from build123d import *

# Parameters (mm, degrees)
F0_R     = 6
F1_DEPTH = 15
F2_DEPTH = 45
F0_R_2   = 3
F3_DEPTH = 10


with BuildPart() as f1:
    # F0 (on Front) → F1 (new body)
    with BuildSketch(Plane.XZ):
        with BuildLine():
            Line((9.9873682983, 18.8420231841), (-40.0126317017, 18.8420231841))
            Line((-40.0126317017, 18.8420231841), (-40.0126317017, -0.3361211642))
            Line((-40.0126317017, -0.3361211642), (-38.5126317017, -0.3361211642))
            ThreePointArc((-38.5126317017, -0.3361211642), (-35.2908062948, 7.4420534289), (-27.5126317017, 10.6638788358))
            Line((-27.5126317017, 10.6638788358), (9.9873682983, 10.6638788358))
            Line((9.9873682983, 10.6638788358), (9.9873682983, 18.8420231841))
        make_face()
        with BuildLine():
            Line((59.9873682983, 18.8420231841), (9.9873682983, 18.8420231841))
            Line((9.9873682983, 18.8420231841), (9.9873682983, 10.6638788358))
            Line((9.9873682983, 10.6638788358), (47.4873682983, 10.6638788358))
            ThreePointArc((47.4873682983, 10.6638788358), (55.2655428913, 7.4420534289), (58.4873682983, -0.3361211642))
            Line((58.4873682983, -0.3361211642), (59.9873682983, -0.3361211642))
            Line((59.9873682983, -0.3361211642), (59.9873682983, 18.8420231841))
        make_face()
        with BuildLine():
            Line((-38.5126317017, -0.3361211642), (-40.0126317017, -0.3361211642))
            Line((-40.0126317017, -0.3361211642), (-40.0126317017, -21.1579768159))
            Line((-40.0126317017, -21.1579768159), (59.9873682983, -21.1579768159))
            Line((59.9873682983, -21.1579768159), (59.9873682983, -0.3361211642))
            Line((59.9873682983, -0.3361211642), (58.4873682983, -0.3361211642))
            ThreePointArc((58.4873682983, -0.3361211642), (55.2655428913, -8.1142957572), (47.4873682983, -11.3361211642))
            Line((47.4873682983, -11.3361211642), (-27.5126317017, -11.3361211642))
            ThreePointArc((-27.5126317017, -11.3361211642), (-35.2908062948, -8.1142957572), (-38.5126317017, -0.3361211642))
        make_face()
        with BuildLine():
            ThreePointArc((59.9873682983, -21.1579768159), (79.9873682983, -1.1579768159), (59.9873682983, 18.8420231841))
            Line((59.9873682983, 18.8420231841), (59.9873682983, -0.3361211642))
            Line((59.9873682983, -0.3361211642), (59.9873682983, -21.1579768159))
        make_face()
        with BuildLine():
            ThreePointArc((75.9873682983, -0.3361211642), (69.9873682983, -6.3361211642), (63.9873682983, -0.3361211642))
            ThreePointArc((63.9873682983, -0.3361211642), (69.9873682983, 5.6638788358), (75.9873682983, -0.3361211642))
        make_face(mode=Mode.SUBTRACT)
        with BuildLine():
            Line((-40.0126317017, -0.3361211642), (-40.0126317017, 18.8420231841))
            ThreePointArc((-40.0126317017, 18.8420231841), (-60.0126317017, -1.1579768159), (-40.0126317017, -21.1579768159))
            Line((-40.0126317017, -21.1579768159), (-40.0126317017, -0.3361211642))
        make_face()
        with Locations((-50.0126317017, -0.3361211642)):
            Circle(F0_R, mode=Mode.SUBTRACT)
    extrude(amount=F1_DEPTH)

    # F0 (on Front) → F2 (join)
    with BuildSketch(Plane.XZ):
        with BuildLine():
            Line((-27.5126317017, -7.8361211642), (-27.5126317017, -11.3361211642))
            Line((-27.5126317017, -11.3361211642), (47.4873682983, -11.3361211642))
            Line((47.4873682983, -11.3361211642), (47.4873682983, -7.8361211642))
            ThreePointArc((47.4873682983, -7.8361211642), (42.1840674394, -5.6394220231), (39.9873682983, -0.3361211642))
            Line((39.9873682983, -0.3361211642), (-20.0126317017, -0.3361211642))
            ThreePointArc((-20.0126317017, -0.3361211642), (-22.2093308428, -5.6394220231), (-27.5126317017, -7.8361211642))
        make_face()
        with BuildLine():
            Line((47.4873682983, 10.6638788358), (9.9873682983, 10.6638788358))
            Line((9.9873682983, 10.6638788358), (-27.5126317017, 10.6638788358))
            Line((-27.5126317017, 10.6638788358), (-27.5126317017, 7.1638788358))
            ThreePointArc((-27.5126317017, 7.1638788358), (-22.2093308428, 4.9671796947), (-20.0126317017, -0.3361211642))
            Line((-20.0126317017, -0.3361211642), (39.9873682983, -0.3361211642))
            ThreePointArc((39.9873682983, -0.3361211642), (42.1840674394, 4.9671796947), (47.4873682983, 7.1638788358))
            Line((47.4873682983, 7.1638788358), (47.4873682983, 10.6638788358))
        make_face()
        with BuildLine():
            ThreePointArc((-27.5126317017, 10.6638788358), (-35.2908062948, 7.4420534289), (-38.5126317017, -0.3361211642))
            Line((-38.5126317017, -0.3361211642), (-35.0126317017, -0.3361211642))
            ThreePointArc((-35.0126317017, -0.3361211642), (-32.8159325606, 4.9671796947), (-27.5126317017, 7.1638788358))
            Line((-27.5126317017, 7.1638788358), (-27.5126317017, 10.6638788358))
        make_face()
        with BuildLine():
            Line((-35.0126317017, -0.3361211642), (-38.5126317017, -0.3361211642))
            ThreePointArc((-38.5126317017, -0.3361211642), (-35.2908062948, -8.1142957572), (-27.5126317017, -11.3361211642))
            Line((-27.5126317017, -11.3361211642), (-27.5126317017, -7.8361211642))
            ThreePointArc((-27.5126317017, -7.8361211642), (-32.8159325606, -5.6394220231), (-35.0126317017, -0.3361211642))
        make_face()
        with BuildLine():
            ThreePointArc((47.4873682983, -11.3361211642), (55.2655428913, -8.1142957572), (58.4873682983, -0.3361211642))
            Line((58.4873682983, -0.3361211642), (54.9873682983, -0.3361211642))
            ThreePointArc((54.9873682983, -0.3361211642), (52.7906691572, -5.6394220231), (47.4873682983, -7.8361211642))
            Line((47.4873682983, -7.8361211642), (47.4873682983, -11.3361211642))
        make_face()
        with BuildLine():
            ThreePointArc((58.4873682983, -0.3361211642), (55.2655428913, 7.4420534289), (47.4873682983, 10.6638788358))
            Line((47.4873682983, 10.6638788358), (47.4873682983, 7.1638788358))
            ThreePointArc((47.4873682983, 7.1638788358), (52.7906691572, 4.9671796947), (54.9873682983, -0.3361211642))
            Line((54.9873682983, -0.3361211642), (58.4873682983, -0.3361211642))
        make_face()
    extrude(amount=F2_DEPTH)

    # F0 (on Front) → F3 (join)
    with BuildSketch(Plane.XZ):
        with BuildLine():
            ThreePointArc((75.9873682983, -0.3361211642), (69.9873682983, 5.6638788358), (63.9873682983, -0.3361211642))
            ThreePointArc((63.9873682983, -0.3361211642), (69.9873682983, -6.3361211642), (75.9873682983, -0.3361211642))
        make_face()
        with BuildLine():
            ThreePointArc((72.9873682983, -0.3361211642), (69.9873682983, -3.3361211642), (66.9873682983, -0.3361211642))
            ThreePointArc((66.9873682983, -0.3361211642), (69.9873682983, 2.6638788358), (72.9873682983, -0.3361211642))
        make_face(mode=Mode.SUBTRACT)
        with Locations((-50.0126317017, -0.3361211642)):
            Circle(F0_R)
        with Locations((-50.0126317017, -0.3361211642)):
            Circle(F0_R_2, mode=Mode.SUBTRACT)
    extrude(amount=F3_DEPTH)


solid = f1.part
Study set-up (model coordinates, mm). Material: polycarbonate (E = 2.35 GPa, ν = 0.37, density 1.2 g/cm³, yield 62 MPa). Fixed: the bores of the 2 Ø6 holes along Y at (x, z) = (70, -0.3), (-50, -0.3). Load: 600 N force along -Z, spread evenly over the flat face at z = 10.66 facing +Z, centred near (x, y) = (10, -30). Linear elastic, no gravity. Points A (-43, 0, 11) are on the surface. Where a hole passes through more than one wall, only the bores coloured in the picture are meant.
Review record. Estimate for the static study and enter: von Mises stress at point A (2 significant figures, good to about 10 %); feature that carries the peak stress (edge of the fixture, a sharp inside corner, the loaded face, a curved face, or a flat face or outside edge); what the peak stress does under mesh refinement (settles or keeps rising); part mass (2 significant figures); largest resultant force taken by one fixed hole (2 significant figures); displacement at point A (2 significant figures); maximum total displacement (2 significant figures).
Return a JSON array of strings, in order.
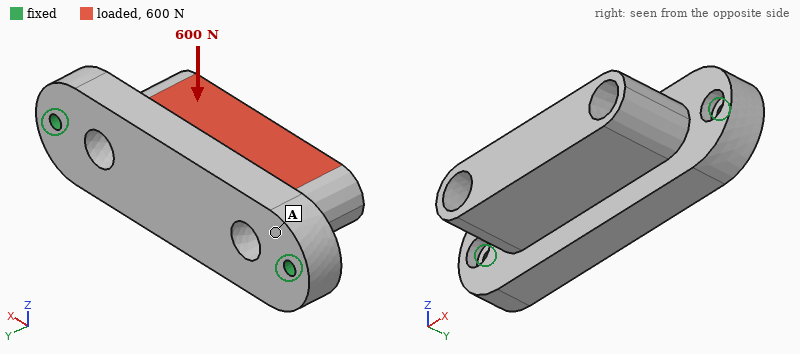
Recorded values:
["2.7 MPa", "edge of the fixture", "keeps rising", "150 g", "300 N", "0.091 mm", "0.60 mm"]
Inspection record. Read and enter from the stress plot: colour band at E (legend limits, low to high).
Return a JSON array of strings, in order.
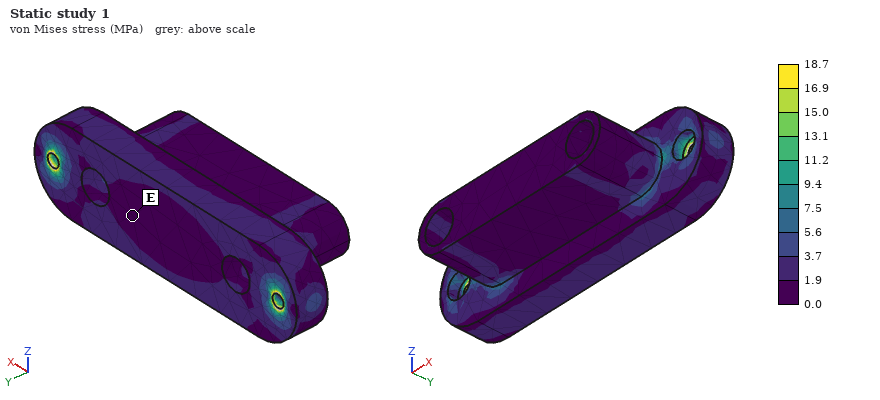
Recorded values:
["0.0 to 1.9 MPa"]
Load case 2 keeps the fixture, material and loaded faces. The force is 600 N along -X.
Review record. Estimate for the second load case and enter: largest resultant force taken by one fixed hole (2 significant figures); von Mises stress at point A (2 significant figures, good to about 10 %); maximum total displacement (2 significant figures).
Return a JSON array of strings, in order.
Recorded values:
["330 N", "0.64 MPa", "47 µm"]
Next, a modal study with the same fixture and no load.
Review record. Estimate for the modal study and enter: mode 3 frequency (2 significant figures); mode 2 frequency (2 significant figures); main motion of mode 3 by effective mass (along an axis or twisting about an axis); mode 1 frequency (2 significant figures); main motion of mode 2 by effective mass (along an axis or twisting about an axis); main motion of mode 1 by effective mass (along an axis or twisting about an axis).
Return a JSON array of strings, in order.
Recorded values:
["1600 Hz", "1300 Hz", "along Z", "700 Hz", "along Y", "along Z"]
